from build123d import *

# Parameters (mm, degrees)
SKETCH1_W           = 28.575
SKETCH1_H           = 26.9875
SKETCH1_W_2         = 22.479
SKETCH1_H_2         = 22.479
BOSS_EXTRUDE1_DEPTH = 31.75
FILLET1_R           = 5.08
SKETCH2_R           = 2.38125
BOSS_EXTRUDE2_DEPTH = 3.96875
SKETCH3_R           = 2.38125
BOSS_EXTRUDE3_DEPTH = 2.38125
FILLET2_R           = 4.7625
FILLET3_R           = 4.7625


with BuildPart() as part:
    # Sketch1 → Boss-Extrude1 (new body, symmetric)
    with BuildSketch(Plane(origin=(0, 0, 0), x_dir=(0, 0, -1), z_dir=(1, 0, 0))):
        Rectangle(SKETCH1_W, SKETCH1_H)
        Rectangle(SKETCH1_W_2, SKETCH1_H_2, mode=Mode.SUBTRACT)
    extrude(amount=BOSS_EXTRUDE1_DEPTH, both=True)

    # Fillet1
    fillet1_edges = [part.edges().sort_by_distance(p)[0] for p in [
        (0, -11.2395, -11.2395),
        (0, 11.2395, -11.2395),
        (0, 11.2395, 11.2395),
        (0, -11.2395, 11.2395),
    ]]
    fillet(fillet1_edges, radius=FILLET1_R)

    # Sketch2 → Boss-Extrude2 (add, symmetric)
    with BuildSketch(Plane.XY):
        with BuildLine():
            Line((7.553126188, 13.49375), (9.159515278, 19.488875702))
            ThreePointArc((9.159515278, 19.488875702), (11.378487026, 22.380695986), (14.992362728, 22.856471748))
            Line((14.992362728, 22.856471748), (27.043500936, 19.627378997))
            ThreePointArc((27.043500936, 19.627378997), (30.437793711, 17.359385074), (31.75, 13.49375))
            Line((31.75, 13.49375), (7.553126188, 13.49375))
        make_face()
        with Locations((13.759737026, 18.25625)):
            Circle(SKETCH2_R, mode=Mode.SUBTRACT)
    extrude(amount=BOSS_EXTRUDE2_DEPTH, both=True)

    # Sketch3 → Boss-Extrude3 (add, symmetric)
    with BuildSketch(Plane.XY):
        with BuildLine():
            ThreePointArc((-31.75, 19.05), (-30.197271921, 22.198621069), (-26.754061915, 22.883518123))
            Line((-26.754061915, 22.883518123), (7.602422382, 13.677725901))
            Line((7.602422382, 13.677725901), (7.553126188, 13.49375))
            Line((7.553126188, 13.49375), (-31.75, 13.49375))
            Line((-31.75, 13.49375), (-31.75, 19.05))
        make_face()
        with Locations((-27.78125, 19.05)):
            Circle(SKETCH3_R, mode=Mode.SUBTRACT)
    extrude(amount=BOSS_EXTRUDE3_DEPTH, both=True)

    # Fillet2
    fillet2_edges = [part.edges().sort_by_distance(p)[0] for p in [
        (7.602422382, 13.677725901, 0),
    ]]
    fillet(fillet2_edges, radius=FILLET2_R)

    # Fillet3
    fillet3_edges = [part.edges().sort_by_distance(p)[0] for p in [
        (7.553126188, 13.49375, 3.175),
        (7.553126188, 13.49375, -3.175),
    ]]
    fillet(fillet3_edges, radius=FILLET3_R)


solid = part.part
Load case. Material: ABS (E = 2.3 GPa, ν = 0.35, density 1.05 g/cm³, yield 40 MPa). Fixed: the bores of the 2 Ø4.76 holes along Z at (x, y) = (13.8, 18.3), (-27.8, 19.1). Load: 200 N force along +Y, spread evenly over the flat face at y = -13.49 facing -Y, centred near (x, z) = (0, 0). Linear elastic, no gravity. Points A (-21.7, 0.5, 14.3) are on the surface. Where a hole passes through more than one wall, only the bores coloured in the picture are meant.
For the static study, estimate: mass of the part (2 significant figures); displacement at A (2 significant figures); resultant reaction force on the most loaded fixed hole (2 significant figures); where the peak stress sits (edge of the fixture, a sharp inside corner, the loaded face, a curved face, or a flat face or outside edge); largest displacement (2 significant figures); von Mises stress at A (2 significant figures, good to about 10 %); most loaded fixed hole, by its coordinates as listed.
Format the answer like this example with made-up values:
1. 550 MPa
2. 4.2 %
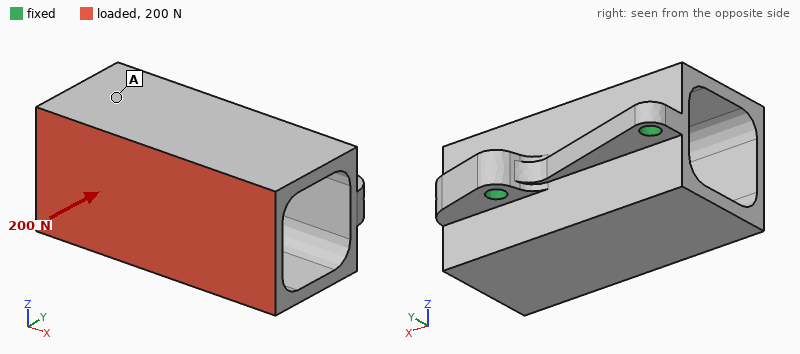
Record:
1. 21 g
2. 0.15 mm
3. 130 N
4. a flat face or outside edge
5. 0.24 mm
6. 3.1 MPa
7. (13.8, 18.3)
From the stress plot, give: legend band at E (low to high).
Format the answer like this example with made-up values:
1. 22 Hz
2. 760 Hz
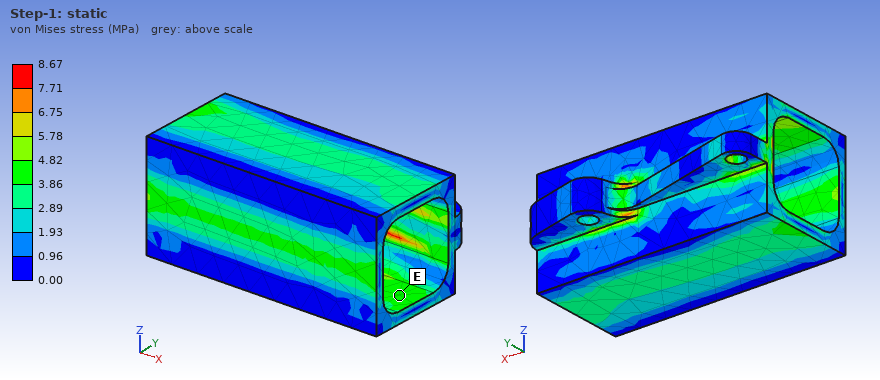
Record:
1. 3.86 to 4.82 MPa
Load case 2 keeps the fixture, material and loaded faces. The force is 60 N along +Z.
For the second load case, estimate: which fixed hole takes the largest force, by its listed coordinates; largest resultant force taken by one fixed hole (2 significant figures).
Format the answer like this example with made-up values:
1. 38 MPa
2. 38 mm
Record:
1. (13.8, 18.3)
2. 48 N
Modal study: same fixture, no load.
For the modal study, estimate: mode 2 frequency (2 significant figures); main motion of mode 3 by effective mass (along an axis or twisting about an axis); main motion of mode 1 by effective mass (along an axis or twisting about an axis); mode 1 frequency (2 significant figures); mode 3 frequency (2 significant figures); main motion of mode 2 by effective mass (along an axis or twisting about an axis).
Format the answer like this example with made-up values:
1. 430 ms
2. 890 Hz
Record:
1. 1400 Hz
2. along Y
3. along Z
4. 440 Hz
5. 1600 Hz
6. along X
